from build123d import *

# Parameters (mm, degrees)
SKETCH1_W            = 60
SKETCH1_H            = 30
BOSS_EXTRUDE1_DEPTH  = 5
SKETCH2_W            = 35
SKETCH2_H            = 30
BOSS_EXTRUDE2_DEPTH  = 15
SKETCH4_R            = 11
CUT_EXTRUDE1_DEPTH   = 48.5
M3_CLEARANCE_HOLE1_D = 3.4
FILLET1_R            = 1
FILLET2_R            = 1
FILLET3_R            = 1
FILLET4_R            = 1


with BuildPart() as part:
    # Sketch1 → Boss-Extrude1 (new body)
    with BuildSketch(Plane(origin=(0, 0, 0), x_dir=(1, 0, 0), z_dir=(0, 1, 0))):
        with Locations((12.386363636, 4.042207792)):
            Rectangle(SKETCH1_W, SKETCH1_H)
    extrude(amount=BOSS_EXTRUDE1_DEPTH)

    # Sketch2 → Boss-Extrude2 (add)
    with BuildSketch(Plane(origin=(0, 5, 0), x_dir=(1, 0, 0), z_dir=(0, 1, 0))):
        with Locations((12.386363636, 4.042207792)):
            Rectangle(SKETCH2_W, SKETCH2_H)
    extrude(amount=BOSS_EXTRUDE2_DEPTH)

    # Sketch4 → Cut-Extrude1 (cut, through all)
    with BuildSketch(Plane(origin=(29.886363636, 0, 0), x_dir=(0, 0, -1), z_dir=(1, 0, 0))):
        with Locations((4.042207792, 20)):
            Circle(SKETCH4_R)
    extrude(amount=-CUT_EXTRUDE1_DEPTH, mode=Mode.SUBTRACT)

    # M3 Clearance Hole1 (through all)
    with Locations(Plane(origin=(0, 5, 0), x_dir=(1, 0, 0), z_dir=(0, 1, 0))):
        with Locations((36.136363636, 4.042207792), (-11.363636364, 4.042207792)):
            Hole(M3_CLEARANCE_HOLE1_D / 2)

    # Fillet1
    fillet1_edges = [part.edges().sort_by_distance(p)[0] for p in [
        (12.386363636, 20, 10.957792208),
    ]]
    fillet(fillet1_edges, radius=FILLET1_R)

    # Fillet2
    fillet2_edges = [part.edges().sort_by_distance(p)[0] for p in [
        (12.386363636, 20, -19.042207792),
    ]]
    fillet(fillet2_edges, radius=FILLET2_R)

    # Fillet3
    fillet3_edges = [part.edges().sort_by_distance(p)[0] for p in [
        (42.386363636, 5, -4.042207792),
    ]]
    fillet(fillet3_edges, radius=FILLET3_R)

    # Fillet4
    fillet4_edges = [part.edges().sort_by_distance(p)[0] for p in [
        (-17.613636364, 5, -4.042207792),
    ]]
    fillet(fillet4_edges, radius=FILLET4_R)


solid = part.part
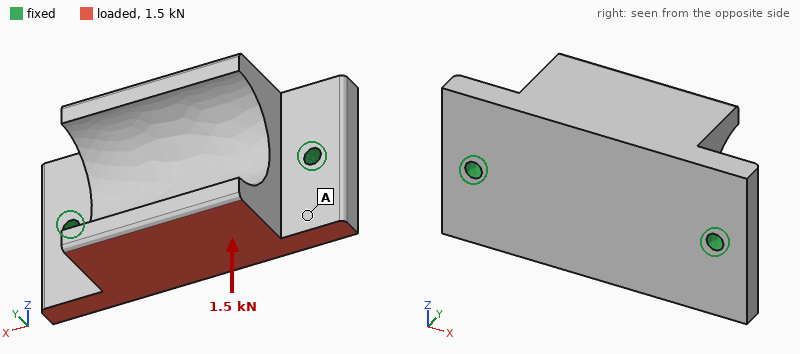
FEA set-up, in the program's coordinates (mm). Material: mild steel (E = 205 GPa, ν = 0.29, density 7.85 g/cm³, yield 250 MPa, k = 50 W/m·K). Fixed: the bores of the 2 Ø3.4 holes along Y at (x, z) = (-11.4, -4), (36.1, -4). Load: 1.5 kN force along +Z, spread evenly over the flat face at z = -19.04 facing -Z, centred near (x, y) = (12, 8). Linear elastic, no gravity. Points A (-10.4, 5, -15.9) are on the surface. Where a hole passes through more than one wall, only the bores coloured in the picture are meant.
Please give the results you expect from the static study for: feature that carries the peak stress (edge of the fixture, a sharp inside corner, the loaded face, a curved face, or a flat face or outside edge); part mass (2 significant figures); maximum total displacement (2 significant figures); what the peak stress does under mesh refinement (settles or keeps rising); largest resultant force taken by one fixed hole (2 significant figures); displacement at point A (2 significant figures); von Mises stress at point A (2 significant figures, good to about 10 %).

edge of the fixture
140 g
15 µm
keeps rising
750 N
5.0 µm
11 MPa
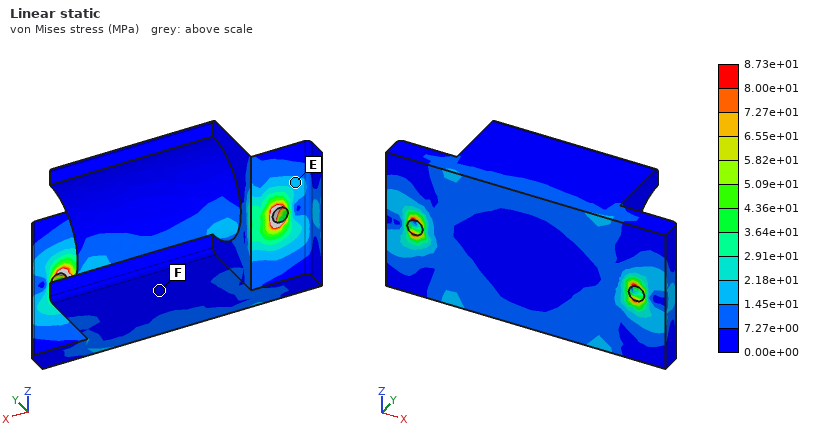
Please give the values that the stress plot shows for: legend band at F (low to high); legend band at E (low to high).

0.00e+00 to 7.27e+00 MPa
1.45e+01 to 2.18e+01 MPa
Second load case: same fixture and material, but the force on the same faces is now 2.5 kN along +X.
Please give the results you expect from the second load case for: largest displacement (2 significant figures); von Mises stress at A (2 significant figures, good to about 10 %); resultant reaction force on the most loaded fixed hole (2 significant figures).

3.7 µm
12 MPa
1.5 kN
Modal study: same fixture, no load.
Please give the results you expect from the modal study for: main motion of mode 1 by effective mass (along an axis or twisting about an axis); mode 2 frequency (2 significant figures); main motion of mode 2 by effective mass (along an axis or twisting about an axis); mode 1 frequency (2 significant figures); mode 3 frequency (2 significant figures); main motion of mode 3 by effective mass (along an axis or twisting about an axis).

along Z
9800 Hz
along Y
5000 Hz
16 kHz
along X
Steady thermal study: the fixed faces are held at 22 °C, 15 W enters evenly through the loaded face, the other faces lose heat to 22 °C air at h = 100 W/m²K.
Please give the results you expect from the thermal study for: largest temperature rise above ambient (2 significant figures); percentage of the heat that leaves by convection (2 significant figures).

18 K
31 %
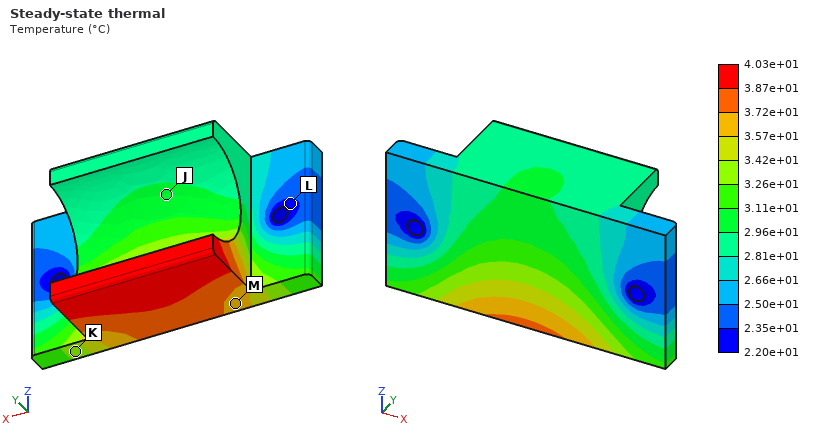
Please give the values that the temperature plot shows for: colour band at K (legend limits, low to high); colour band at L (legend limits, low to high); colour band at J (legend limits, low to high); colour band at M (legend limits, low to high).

3.26e+01 to 3.42e+01 °C
2.20e+01 to 2.35e+01 °C
2.96e+01 to 3.11e+01 °C
3.57e+01 to 3.72e+01 °C
